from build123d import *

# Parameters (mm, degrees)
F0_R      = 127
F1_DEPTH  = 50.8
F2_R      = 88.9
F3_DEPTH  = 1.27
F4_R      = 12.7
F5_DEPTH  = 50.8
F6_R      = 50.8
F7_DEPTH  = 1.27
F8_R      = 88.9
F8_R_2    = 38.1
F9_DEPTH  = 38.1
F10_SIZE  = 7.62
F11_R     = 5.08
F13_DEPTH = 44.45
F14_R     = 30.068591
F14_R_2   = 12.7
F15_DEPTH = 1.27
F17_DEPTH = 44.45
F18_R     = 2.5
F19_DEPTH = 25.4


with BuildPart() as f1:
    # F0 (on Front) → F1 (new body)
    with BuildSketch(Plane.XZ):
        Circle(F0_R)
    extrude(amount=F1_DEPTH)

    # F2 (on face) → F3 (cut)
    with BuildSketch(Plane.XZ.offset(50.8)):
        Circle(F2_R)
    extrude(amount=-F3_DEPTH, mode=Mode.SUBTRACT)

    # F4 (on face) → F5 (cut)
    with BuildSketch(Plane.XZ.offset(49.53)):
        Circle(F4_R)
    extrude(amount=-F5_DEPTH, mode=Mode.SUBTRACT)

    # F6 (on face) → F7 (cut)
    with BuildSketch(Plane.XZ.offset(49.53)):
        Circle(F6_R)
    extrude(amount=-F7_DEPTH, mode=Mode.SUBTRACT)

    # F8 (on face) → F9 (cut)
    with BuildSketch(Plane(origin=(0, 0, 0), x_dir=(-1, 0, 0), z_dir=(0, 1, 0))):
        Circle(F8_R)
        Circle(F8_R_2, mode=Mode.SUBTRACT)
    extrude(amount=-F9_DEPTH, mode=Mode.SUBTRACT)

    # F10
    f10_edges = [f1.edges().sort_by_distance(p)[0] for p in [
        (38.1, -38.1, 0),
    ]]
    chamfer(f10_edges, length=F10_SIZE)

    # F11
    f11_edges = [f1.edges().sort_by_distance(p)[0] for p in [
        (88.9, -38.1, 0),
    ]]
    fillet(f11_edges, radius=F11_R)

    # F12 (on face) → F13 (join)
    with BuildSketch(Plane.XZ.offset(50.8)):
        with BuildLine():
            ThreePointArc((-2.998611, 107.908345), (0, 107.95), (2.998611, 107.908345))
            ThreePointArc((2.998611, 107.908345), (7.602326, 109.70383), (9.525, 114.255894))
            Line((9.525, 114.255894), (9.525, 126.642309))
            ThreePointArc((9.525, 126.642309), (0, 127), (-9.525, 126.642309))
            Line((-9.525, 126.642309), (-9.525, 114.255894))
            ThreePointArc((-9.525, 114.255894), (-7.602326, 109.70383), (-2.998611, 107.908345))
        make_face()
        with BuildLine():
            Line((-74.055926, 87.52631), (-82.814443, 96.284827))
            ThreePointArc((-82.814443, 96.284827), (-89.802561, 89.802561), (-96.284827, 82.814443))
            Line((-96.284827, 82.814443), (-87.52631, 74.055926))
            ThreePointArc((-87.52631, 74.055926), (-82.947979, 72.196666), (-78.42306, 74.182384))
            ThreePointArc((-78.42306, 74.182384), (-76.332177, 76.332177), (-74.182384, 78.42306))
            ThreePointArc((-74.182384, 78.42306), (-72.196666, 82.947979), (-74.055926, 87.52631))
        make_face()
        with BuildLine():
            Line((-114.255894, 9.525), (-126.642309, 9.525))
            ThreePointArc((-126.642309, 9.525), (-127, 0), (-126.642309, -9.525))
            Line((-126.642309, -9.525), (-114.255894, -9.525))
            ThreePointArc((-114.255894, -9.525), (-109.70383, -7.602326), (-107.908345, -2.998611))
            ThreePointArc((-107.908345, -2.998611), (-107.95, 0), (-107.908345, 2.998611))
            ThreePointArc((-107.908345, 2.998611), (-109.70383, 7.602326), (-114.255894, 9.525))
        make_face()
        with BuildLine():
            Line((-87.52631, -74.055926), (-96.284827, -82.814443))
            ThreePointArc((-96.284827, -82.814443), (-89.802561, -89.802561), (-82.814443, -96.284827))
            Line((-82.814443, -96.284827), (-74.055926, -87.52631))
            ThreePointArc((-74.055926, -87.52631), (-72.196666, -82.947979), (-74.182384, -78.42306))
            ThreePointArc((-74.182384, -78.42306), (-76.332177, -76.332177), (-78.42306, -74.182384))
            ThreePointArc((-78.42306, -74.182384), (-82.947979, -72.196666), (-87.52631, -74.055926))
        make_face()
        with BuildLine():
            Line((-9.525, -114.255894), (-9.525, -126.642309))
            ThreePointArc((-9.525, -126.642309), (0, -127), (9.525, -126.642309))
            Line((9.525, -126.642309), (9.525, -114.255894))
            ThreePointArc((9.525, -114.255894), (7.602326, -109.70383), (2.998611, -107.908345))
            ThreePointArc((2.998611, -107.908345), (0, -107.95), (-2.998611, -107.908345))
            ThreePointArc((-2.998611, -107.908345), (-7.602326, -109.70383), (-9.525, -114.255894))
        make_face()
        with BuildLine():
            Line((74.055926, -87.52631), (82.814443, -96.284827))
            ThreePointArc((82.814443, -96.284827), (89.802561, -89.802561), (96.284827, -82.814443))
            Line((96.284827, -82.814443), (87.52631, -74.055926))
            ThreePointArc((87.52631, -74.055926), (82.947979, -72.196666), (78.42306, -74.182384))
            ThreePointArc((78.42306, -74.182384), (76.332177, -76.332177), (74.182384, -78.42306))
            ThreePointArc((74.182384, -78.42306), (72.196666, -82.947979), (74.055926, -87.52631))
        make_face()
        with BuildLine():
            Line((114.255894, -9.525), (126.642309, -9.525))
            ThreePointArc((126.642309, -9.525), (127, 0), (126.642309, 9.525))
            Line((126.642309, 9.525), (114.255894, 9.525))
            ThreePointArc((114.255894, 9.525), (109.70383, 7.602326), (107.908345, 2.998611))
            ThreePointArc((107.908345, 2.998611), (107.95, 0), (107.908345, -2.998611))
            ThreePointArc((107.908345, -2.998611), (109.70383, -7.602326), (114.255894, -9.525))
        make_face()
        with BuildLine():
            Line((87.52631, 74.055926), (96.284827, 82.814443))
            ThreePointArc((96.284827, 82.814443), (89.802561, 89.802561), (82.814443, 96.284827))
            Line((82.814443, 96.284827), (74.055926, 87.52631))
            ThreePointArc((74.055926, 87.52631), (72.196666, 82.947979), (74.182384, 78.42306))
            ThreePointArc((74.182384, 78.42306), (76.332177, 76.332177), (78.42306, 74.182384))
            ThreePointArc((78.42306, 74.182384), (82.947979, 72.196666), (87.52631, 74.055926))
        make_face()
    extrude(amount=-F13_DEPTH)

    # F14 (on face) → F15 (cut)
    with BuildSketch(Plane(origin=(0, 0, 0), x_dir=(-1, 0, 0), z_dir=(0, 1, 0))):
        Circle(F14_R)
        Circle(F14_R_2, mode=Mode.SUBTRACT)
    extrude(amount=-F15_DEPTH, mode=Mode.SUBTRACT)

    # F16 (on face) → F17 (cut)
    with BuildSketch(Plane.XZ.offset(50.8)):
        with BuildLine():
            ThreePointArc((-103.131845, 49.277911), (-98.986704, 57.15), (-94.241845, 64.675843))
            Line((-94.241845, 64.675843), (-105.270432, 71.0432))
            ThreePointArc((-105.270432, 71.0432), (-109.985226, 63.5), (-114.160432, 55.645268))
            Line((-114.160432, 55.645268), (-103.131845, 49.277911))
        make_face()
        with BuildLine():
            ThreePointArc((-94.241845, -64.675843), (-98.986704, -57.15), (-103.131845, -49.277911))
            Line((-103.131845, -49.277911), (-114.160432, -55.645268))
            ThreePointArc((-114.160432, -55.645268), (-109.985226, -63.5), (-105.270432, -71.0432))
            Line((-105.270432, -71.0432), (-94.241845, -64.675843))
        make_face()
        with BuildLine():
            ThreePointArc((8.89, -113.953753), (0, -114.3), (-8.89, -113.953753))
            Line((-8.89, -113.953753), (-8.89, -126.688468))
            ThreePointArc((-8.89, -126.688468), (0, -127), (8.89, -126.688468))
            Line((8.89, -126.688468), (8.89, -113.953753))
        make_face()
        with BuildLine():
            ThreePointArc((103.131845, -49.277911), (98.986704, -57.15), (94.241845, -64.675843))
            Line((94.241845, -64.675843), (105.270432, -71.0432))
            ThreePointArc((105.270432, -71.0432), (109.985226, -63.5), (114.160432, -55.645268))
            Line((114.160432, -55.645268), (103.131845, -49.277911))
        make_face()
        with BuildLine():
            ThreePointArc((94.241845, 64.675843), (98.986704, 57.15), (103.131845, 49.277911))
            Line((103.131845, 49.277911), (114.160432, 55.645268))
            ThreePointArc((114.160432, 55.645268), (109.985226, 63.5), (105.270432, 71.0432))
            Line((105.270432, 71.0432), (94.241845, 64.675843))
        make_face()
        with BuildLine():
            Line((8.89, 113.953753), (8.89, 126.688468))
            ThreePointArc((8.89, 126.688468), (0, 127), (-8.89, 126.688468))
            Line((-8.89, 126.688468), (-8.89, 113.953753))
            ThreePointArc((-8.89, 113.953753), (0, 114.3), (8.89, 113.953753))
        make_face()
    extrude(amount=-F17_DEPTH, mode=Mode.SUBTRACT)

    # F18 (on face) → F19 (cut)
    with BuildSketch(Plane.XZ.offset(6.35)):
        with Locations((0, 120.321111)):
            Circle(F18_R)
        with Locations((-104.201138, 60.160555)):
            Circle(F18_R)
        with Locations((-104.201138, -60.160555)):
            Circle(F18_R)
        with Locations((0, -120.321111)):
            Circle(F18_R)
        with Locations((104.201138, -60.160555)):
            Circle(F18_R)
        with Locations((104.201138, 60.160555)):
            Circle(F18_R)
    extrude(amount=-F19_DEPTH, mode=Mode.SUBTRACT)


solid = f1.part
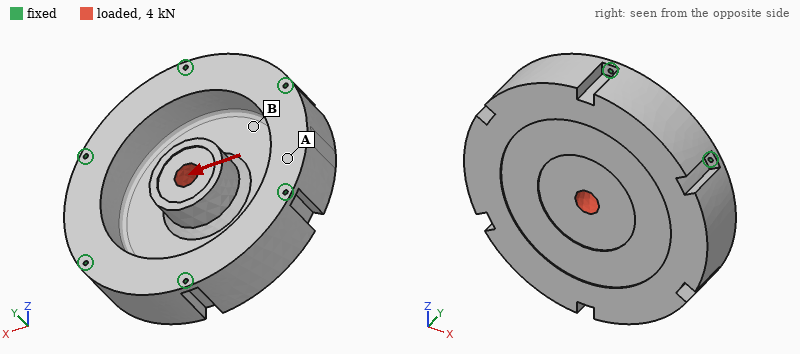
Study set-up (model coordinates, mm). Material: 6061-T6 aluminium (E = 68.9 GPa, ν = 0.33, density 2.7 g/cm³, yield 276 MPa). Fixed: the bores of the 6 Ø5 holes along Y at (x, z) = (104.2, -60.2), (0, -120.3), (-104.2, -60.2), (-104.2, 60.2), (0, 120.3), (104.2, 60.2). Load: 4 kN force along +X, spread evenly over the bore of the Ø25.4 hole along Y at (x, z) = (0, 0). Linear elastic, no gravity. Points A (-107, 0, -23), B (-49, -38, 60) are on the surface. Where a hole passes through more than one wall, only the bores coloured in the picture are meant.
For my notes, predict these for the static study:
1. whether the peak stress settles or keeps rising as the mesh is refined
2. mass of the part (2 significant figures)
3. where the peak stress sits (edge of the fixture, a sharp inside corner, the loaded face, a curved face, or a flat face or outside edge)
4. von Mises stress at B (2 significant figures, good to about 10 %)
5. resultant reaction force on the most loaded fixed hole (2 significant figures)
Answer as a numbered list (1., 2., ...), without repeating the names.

1. keeps rising
2. 4.5 kg
3. edge of the fixture
4. 1.9 MPa
5. 980 N
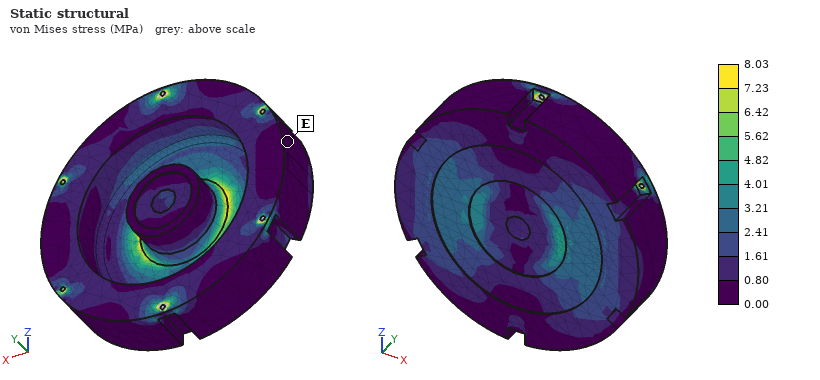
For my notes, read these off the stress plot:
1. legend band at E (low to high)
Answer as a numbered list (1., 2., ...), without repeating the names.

1. 0.00 to 0.80 MPa
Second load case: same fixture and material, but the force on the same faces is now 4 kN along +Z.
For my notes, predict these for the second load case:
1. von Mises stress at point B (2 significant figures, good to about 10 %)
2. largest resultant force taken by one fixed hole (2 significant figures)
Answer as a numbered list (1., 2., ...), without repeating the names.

1. 1.6 MPa
2. 880 N
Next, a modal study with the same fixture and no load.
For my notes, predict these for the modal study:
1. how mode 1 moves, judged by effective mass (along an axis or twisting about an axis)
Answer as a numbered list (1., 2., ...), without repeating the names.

1. along Y
